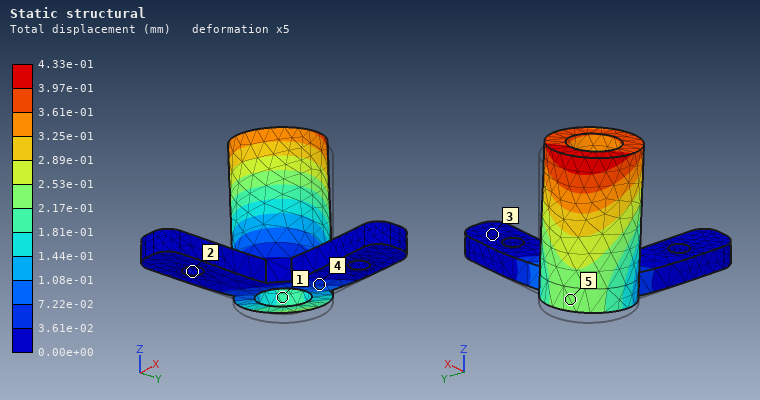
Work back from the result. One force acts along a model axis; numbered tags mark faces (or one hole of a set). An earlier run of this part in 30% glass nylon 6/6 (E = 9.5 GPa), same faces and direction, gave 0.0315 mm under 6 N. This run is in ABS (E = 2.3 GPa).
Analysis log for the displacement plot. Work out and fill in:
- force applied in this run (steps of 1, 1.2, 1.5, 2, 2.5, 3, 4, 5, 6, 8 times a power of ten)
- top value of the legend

20 N
4.33e-01 mm
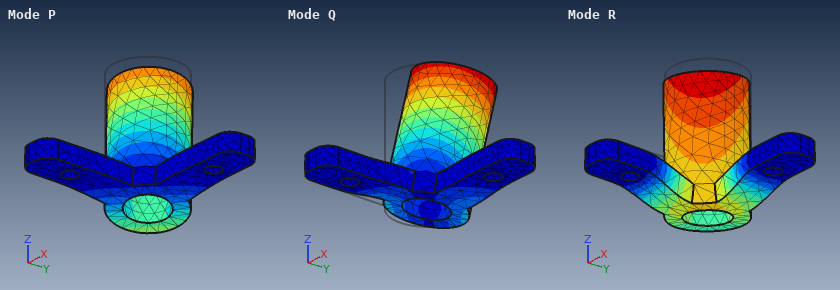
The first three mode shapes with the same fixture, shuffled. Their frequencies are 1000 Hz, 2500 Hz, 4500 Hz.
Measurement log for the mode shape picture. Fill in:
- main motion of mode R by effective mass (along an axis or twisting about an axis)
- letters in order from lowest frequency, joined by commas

along Z
P, Q, R
